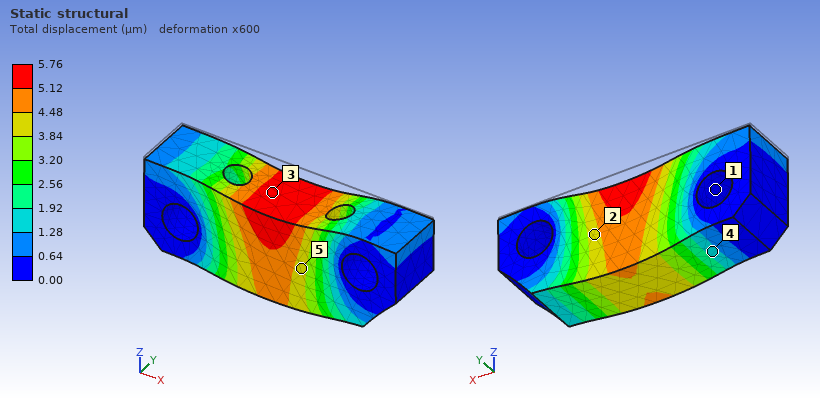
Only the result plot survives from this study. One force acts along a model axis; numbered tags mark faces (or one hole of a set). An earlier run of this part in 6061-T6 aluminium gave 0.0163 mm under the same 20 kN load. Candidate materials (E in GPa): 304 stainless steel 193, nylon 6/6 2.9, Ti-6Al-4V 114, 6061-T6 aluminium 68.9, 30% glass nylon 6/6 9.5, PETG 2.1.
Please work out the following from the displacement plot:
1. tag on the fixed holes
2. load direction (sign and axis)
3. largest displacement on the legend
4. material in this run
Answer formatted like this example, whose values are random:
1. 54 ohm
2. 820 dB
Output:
1. 1
2. -Z
3. 5.76 µm
4. 304 stainless steel
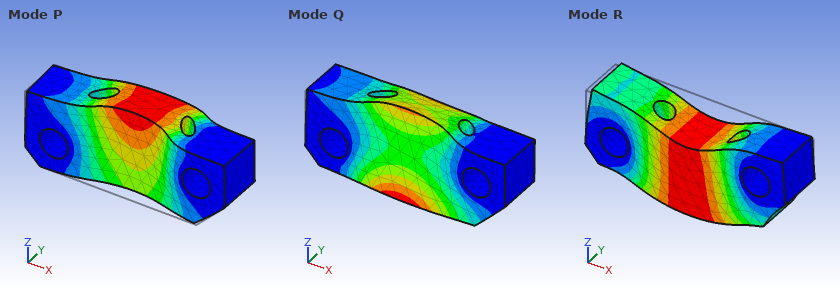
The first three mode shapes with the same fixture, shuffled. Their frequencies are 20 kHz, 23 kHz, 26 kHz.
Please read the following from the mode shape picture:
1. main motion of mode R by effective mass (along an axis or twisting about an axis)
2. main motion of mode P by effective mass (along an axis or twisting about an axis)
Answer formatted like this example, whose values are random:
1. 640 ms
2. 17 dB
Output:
1. along Z
2. along Y
